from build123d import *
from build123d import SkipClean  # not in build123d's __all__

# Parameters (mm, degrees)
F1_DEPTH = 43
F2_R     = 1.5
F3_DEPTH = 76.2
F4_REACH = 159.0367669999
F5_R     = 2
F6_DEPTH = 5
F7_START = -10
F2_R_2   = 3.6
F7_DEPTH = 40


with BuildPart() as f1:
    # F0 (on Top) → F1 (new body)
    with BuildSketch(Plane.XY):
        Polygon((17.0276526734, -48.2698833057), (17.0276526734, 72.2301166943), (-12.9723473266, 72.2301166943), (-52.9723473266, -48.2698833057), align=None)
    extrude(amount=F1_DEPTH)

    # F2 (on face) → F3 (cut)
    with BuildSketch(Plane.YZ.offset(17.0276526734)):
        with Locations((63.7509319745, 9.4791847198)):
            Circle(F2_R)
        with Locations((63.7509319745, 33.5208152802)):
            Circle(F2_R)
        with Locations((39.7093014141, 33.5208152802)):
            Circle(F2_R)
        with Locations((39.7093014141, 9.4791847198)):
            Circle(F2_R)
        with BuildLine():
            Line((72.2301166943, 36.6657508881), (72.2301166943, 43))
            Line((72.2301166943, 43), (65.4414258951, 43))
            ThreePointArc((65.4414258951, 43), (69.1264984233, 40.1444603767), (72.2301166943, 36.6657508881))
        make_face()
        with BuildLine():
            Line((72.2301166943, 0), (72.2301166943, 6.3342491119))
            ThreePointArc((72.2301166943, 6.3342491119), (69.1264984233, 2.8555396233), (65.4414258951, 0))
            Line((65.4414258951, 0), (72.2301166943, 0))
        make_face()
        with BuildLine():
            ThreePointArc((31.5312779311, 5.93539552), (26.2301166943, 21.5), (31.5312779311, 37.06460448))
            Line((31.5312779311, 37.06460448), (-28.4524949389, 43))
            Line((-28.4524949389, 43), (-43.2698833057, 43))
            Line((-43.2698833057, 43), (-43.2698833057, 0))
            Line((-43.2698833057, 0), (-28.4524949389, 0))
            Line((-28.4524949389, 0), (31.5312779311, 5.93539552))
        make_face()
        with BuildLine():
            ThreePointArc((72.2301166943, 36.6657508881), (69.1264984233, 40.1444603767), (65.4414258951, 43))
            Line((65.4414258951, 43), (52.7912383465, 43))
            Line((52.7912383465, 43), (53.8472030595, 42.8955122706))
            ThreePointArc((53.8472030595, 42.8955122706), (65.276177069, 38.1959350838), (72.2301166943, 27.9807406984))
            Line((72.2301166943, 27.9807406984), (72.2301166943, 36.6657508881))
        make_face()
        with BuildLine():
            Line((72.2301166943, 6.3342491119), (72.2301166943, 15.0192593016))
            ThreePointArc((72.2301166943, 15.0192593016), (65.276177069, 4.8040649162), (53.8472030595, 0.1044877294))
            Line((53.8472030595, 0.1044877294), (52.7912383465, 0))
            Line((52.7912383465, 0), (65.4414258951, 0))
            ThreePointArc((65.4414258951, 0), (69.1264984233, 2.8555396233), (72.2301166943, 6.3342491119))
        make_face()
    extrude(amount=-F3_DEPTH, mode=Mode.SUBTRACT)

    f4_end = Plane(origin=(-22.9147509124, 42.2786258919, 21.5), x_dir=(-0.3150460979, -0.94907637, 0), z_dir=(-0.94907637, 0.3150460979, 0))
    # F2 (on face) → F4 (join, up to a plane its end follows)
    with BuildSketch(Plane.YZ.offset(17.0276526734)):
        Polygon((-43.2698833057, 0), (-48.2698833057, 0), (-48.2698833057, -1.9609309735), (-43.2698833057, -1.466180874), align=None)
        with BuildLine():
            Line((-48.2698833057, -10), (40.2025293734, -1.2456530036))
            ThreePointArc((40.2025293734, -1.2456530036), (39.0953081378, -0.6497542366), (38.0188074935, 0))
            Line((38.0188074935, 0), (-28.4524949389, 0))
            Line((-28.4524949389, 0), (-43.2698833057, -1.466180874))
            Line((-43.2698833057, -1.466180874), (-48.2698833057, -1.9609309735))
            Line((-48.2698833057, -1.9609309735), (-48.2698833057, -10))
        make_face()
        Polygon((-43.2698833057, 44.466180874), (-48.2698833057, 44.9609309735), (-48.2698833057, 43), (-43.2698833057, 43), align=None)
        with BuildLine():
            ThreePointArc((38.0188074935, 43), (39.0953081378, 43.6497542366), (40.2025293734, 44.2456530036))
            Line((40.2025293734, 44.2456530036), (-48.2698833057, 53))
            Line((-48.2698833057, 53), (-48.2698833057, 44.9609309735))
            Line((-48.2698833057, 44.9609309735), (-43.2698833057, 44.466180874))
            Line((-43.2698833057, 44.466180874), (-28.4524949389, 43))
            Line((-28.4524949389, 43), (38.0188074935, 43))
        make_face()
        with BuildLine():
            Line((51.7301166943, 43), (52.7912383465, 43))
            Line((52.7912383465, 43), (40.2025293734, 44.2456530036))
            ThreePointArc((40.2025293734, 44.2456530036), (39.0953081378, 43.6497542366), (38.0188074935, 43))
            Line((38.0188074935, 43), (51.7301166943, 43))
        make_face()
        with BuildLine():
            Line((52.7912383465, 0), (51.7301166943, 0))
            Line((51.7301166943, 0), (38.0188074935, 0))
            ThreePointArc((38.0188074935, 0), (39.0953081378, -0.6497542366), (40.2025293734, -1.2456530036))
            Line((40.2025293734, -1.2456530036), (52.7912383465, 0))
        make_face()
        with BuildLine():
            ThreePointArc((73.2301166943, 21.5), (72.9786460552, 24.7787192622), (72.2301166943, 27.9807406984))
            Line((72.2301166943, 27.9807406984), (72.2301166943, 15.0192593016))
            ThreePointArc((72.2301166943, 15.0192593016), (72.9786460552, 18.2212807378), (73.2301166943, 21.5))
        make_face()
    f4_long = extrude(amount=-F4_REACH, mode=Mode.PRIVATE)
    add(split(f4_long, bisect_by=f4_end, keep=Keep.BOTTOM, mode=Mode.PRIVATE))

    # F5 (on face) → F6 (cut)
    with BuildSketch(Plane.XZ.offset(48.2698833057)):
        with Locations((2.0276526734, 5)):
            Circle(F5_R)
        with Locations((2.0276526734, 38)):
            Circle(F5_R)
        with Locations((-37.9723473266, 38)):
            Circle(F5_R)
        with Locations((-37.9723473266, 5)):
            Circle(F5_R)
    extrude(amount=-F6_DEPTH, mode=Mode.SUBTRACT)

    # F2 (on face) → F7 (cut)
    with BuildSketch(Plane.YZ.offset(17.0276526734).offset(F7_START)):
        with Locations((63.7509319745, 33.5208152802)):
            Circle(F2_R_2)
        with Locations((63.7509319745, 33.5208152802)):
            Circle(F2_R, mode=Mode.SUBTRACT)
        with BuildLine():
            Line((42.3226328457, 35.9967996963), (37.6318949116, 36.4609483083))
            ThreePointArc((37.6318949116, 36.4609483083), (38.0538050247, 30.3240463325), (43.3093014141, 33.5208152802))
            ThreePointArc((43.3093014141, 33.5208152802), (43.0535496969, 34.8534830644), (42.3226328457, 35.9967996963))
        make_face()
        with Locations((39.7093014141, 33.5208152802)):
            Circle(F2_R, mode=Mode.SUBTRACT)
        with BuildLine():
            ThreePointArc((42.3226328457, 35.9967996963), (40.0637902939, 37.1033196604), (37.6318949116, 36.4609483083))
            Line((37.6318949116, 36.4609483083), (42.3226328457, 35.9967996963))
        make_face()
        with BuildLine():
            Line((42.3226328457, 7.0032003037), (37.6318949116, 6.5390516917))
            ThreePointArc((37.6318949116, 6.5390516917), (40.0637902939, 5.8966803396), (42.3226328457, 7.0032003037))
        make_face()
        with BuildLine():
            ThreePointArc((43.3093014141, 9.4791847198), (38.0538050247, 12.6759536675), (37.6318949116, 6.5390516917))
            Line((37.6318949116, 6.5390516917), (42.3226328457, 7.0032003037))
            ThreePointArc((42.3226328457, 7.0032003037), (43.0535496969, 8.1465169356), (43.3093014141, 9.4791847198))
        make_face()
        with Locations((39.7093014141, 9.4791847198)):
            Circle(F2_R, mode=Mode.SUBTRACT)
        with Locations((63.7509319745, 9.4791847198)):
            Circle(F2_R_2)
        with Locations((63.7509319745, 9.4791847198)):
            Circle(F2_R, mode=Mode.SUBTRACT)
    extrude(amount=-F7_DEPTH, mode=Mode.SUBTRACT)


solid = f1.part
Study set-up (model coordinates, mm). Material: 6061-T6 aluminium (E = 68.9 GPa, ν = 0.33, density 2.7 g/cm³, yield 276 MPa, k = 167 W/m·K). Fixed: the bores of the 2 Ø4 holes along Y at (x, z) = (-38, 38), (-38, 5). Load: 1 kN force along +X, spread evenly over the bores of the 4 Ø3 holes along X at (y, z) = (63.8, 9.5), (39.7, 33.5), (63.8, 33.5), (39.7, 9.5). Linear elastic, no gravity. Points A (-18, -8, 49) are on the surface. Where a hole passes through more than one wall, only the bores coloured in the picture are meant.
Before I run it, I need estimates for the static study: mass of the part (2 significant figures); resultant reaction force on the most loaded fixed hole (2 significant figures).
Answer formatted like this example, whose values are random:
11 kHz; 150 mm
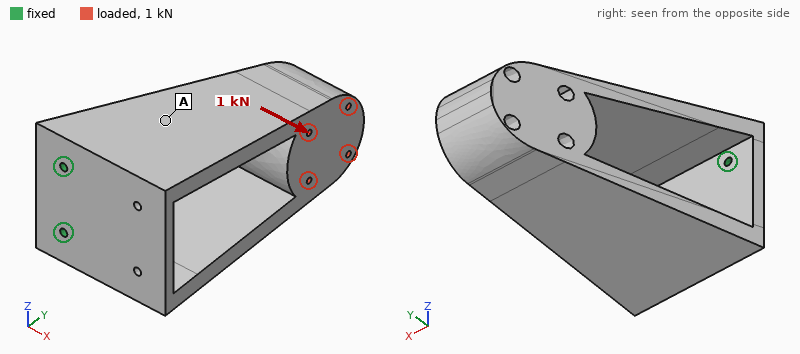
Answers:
410 g; 510 N
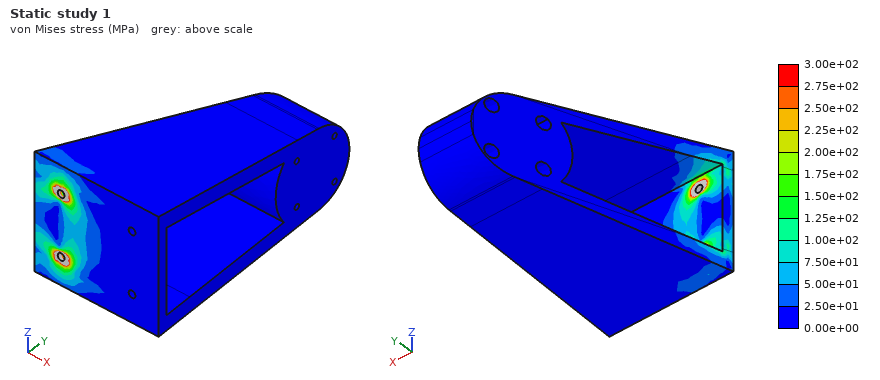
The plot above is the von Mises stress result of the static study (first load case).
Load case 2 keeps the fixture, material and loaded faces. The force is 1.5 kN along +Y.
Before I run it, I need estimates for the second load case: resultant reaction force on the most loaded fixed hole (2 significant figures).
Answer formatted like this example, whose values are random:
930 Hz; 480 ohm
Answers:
760 N
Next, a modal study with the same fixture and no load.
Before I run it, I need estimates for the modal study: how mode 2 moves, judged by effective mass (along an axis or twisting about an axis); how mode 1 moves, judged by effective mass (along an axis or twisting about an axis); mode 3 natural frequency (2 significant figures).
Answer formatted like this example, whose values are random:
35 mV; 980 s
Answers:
along Z; along X; 2400 Hz
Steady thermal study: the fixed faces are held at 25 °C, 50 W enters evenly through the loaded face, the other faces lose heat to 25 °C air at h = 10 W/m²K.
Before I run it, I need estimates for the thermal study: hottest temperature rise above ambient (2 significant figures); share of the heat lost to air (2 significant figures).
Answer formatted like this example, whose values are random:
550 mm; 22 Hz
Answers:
45 K; 19 %
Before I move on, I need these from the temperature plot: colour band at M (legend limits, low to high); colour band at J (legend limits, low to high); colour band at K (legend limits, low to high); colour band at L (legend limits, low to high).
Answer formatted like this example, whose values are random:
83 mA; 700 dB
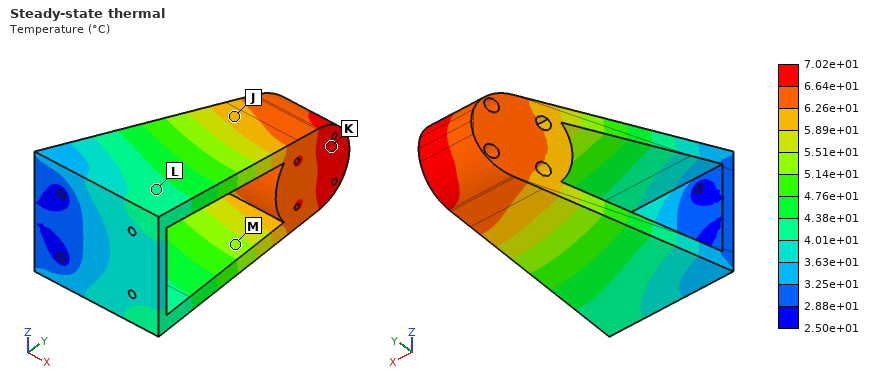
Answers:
5.14e+01 to 5.51e+01 °C; 5.89e+01 to 6.26e+01 °C; 6.64e+01 to 7.02e+01 °C; 4.01e+01 to 4.38e+01 °C
